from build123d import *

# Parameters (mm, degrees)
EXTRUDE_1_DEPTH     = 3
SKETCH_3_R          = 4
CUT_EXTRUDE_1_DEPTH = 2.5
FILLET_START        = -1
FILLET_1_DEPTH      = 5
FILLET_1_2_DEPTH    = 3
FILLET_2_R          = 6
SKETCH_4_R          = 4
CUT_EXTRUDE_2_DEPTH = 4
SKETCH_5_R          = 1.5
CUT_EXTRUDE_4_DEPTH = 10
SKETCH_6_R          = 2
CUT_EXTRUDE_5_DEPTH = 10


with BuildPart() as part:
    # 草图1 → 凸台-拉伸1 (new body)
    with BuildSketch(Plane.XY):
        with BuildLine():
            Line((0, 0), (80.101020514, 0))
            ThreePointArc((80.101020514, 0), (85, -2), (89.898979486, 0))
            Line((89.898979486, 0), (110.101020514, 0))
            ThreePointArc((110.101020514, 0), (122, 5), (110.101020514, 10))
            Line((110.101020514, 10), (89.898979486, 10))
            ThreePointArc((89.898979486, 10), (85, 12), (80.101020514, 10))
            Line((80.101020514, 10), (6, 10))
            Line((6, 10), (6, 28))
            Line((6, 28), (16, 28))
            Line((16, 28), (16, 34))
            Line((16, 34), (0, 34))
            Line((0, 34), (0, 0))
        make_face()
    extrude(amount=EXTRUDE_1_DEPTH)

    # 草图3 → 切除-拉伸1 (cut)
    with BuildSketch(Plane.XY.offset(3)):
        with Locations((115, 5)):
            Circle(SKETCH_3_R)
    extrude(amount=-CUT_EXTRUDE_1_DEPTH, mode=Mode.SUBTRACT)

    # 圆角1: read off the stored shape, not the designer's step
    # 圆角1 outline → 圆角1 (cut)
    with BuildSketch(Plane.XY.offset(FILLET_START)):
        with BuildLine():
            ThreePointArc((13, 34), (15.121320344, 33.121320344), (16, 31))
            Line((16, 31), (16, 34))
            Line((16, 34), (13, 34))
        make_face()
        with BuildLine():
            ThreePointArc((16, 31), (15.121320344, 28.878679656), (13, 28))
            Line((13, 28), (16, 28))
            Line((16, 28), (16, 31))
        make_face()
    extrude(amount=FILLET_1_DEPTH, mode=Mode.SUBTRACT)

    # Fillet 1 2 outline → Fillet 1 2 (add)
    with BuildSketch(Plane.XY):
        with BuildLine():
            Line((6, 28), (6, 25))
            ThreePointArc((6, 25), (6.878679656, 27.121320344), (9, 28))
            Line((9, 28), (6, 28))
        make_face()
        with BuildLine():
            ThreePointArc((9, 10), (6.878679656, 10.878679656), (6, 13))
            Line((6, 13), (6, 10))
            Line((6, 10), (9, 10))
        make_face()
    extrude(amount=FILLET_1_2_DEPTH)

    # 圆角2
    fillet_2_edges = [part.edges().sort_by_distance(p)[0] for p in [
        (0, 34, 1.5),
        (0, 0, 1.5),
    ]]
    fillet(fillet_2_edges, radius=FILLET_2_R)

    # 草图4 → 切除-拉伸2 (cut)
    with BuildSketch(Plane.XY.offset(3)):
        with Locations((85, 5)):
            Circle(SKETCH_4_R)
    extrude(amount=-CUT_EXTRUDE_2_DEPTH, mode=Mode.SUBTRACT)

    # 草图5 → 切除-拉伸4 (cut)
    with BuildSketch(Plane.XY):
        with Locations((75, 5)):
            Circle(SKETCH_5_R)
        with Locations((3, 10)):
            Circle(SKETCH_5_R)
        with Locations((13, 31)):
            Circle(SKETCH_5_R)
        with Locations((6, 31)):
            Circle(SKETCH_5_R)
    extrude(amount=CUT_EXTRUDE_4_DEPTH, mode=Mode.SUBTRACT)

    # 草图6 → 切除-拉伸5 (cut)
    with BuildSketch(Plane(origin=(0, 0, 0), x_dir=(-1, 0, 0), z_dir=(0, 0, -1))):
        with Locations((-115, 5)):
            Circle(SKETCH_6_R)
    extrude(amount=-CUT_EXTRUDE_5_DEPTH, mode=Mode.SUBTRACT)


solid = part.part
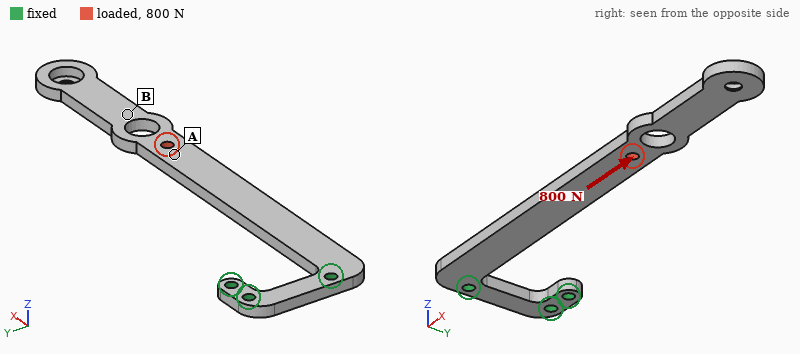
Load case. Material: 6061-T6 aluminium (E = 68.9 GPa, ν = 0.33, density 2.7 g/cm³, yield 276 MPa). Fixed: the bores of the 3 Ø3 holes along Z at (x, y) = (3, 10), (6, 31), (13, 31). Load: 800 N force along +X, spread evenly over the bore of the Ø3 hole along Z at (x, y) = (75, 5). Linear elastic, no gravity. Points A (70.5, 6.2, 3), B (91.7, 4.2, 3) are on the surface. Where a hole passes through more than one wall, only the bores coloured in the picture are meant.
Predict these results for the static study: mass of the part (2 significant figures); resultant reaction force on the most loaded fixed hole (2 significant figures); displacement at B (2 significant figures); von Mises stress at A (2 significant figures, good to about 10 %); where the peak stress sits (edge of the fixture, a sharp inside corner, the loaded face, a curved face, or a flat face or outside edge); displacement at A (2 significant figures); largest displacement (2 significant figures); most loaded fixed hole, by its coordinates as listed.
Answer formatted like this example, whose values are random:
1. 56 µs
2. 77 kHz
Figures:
1. 11 g
2. 840 N
3. 0.25 mm
4. 30 MPa
5. edge of the fixture
6. 0.19 mm
7. 0.33 mm
8. (3, 10)
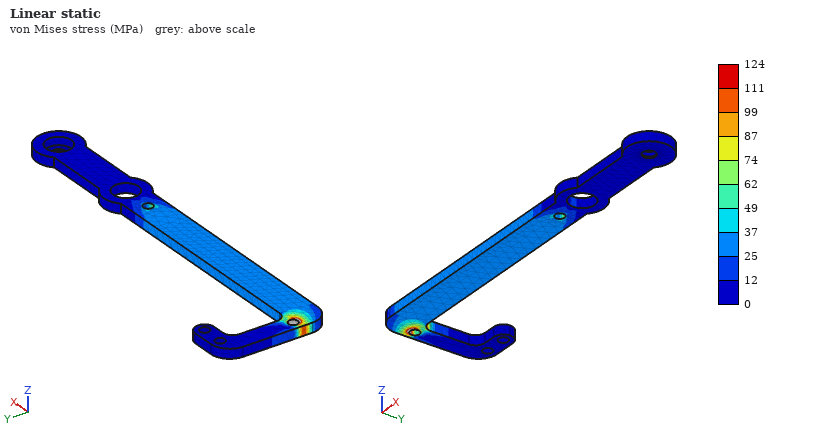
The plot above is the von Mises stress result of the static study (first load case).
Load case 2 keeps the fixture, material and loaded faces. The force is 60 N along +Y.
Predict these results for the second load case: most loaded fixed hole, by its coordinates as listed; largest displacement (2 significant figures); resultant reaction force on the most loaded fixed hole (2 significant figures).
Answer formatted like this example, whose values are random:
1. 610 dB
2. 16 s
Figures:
1. (3, 10)
2. 1.2 mm
3. 73 N
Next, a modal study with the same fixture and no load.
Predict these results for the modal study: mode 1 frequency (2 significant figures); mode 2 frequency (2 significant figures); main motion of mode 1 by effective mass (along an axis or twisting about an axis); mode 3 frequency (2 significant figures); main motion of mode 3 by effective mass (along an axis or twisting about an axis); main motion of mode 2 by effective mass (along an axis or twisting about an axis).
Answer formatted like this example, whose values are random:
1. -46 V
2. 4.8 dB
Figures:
1. 180 Hz
2. 520 Hz
3. along Z
4. 1000 Hz
5. along Z
6. along Y
